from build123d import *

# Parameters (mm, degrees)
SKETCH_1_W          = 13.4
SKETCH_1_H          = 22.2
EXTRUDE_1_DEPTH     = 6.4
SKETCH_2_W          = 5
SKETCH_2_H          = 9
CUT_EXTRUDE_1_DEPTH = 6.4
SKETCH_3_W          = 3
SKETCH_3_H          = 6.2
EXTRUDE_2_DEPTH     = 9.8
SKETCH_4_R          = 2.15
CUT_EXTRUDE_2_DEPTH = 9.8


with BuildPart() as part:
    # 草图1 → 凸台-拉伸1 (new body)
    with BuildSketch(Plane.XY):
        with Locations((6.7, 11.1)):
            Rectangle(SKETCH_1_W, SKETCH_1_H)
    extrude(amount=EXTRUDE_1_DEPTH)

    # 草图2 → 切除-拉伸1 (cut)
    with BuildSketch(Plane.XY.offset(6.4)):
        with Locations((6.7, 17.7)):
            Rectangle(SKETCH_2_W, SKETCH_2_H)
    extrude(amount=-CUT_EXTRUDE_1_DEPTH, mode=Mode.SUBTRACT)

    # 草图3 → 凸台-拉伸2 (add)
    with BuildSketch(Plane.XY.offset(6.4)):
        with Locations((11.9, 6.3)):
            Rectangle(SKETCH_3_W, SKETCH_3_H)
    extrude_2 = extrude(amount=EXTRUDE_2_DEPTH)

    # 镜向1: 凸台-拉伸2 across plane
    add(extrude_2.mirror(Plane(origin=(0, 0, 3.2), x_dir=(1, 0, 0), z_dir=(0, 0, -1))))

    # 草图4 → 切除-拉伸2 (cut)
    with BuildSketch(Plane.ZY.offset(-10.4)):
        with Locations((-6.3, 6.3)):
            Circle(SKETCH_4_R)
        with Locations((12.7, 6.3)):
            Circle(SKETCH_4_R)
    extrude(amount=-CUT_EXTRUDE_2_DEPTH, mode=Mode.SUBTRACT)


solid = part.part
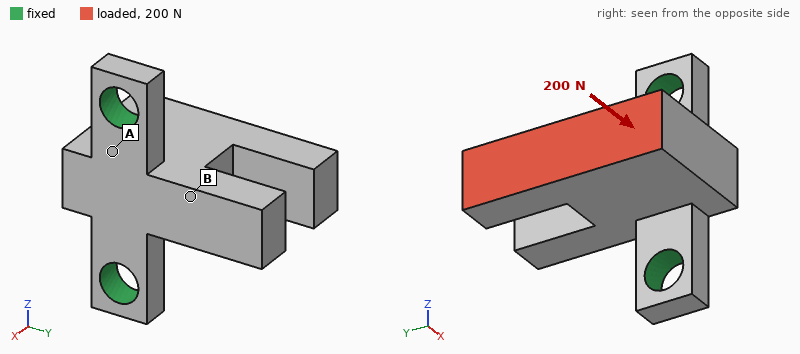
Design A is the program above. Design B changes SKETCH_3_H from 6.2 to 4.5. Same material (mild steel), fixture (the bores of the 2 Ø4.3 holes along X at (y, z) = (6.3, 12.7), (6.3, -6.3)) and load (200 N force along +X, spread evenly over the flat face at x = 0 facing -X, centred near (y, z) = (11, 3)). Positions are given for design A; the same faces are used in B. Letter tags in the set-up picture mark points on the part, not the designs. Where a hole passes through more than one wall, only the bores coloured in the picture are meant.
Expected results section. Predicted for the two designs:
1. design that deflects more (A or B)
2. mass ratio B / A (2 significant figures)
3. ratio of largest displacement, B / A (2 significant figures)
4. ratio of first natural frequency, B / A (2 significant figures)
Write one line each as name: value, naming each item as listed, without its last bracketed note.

design that deflects more: B
mass ratio B / A: 0.95
ratio of largest displacement, B / A: 1.6
ratio of first natural frequency, B / A: 0.76
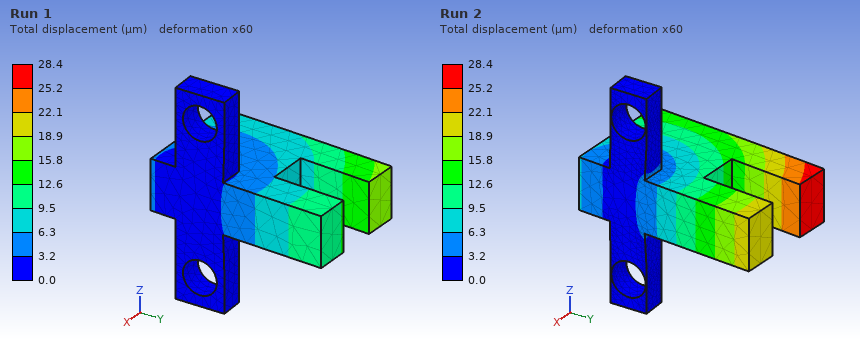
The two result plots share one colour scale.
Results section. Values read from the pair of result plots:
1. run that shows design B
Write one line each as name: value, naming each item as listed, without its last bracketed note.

run that shows design B: Run 2
